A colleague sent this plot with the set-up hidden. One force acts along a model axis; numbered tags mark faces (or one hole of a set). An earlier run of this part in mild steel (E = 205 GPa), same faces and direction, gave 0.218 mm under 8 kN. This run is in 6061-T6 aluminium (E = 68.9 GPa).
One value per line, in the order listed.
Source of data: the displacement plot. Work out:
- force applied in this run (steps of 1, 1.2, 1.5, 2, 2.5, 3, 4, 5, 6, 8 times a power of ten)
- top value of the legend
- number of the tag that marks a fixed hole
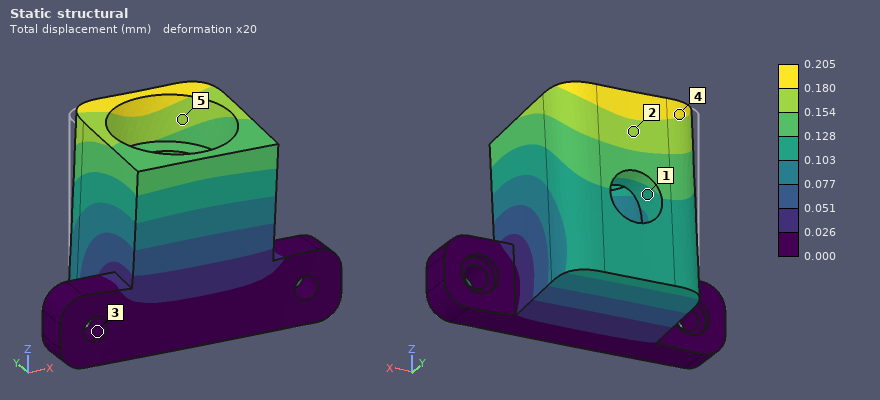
2.5 kN
0.205 mm
3
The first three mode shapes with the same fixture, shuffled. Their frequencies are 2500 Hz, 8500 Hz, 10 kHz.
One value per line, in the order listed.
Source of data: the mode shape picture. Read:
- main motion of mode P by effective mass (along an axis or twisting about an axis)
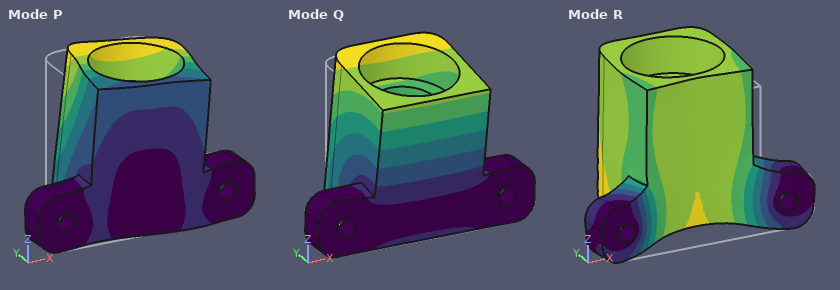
along X
